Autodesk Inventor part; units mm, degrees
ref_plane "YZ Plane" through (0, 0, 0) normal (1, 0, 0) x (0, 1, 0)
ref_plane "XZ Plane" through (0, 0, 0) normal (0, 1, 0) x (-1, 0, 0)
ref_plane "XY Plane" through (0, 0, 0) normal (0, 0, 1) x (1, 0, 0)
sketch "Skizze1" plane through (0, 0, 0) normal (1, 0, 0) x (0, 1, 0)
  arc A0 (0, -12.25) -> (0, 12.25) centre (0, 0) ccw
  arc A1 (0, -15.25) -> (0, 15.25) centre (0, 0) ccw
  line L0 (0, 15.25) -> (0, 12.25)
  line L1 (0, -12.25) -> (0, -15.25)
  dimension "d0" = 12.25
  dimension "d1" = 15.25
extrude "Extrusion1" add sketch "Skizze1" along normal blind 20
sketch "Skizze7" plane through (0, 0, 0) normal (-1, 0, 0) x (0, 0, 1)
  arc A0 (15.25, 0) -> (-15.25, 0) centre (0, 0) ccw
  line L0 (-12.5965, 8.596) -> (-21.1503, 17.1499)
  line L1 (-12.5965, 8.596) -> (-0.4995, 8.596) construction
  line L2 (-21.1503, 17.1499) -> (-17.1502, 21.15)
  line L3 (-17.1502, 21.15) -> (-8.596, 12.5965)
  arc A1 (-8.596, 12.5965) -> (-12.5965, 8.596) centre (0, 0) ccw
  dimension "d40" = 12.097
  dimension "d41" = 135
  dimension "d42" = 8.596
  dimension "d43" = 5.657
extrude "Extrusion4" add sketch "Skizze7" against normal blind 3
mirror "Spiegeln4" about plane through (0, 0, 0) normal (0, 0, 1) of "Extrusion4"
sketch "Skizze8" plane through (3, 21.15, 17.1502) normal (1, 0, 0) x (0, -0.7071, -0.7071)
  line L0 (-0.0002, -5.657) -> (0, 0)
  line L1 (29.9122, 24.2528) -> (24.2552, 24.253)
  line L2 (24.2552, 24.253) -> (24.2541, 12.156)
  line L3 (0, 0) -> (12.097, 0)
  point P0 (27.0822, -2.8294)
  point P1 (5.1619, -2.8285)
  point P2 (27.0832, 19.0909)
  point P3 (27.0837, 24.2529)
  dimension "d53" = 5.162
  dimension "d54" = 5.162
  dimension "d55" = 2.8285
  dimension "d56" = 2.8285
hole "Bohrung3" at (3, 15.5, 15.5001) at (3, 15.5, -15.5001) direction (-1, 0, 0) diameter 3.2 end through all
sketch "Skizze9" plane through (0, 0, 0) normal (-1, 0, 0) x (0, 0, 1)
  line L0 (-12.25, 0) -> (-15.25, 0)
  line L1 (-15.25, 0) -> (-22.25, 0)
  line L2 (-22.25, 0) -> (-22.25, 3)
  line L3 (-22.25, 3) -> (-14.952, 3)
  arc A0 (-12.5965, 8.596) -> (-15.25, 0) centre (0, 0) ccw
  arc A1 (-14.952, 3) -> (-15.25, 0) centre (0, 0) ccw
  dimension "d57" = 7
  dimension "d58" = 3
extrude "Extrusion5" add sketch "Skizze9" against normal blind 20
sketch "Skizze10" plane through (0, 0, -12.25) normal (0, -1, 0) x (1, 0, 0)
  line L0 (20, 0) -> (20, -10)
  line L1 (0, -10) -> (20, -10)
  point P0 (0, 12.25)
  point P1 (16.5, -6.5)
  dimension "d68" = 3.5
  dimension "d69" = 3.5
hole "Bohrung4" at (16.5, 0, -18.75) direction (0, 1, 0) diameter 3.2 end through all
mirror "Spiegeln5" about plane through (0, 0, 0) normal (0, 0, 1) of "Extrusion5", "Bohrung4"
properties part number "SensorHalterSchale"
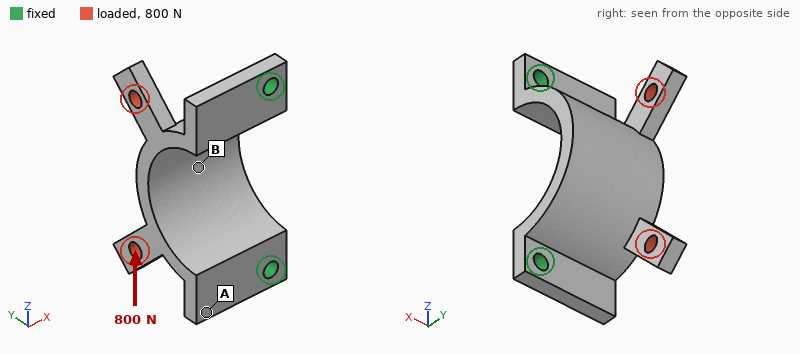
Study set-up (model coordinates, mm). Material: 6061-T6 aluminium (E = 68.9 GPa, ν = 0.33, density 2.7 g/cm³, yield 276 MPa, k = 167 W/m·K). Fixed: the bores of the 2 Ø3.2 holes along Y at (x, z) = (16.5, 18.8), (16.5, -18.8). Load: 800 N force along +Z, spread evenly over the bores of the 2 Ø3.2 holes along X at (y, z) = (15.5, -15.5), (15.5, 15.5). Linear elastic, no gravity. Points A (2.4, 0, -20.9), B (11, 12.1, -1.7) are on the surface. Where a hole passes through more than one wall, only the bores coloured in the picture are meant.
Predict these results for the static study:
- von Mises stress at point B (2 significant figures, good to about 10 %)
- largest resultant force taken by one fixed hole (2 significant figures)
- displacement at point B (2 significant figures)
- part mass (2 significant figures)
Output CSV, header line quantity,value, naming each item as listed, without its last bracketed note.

quantity,value
von Mises stress at point B,43 MPa
largest resultant force taken by one fixed hole,590 N
displacement at point B,0.023 mm
part mass,10 g
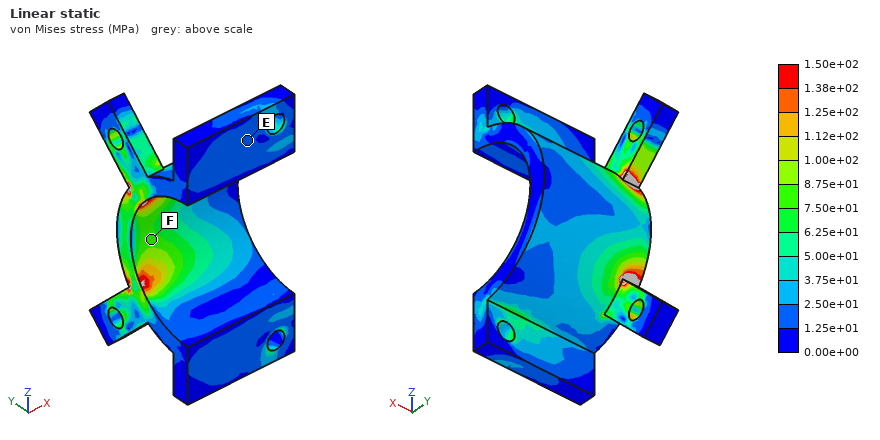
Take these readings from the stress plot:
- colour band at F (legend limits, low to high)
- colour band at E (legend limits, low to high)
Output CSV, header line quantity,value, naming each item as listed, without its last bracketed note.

quantity,value
colour band at F,7.50e+01 to 8.75e+01 MPa
colour band at E,1.25e+01 to 2.50e+01 MPa
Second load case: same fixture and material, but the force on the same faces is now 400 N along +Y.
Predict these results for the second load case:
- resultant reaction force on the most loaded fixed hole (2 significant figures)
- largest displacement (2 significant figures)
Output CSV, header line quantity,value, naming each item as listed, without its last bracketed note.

quantity,value
resultant reaction force on the most loaded fixed hole,200 N
largest displacement,0.15 mm
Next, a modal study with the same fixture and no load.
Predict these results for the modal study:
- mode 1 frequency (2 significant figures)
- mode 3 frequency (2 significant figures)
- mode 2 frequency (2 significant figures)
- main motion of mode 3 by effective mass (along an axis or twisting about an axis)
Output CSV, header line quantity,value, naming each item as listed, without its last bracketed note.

quantity,value
mode 1 frequency,4300 Hz
mode 3 frequency,12 kHz
mode 2 frequency,8200 Hz
main motion of mode 3 by effective mass,along Z
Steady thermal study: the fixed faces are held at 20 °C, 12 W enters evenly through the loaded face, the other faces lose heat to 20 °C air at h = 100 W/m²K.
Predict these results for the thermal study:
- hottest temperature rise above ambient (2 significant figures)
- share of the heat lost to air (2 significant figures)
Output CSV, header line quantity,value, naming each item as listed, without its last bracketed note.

quantity,value
hottest temperature rise above ambient,32 K
share of the heat lost to air,23 %
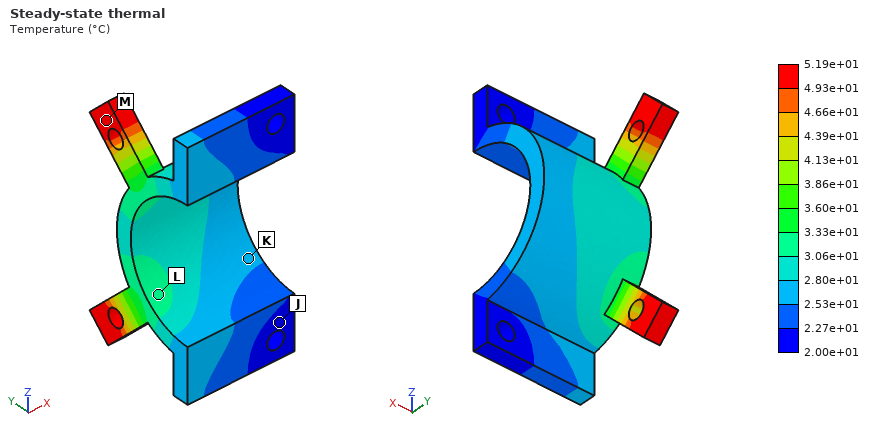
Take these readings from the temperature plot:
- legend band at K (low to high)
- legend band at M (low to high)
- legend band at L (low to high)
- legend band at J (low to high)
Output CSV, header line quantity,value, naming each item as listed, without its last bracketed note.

quantity,value
legend band at K,2.53e+01 to 2.80e+01 °C
legend band at M,4.93e+01 to 5.19e+01 °C
legend band at L,3.06e+01 to 3.33e+01 °C
legend band at J,2.00e+01 to 2.27e+01 °C
